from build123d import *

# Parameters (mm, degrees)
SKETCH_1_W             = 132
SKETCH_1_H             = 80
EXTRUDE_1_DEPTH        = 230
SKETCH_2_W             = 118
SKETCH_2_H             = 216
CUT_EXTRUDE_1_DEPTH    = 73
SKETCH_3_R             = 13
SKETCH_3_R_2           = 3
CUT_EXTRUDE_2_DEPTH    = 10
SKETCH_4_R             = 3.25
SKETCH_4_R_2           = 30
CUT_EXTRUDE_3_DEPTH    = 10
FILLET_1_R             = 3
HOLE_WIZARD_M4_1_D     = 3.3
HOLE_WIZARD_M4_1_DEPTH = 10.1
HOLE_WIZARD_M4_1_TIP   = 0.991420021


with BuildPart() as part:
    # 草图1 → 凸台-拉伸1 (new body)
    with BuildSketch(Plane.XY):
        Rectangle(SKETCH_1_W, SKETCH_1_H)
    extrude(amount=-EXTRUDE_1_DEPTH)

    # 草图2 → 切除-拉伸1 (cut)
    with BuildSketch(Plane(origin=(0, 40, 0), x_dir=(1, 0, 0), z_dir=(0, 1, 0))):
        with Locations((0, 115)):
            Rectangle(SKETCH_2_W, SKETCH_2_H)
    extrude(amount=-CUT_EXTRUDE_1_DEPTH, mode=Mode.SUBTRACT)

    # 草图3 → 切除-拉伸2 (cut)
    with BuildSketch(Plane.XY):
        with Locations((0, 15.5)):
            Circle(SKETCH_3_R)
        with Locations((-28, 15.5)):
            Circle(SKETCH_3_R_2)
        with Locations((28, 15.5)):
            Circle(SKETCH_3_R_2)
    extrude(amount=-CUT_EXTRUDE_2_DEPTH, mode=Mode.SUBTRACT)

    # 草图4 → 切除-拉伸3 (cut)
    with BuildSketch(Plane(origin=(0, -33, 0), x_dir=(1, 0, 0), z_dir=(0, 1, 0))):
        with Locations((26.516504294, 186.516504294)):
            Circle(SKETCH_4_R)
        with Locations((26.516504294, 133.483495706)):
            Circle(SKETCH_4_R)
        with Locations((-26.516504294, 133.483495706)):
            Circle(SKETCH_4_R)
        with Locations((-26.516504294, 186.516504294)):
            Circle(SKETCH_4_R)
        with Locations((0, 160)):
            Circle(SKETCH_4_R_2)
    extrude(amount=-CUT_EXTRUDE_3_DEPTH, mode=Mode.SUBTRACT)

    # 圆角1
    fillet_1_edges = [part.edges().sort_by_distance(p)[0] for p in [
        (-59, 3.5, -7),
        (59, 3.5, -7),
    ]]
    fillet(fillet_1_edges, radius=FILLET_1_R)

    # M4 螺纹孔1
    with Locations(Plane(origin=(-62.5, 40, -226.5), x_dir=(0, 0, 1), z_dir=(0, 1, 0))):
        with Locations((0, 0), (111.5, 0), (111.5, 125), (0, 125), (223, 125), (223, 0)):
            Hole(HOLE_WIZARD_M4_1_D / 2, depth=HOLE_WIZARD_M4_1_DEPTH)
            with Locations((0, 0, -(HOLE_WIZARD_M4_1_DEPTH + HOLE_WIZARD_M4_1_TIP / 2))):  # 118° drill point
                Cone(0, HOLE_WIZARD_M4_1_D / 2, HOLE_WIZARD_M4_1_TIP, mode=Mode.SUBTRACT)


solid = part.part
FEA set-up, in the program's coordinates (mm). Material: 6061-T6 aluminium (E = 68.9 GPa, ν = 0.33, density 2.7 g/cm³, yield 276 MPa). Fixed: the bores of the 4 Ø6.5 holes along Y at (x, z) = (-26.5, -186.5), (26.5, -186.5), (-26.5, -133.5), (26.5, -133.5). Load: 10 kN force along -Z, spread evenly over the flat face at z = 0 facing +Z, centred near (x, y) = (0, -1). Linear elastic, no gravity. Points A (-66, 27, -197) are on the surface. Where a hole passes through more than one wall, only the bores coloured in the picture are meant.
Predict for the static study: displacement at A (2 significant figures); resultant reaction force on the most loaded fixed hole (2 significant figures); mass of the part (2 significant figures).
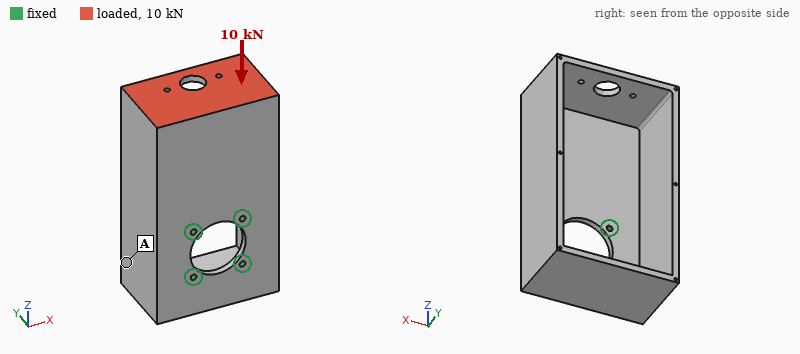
0.25 mm
4.1 kN
1.5 kg
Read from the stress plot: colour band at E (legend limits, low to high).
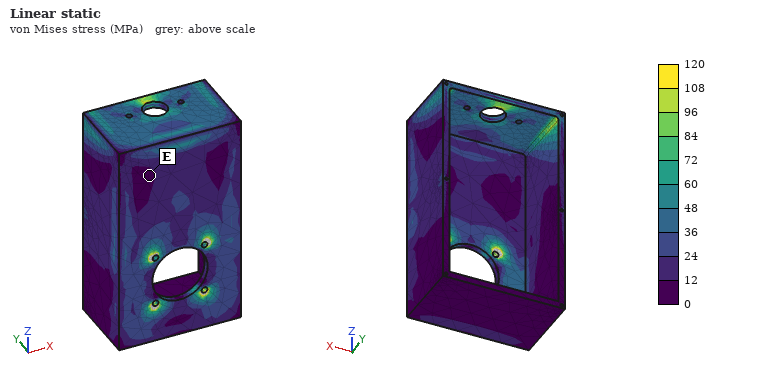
0 to 12 MPa
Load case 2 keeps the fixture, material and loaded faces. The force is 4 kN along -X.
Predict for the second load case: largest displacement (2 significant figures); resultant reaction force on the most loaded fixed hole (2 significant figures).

0.94 mm
6.0 kN
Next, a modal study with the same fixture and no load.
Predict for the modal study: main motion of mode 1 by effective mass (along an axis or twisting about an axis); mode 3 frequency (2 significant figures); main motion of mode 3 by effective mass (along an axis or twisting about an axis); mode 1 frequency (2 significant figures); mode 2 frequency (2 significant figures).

along Y
820 Hz
along X
390 Hz
450 Hz
